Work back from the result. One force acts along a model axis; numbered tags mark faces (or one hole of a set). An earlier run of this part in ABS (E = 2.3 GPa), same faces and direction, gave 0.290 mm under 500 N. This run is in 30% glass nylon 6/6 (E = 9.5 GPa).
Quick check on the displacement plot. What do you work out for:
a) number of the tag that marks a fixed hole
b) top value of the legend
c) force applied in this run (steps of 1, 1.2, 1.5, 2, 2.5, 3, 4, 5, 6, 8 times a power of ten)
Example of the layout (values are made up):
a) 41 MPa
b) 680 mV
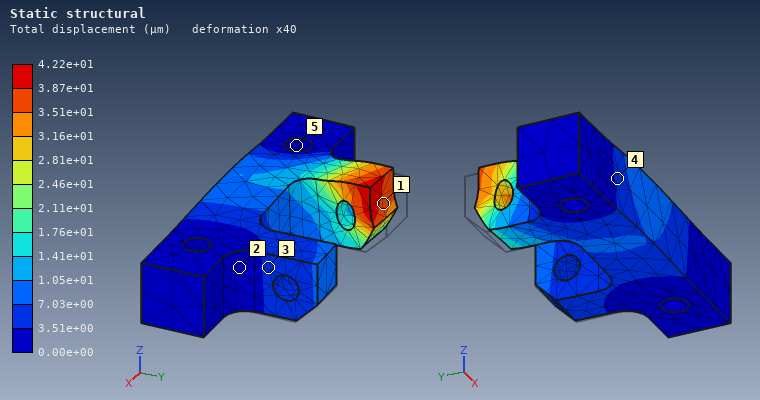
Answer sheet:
a) 5
b) 4.22e+01 µm
c) 300 N
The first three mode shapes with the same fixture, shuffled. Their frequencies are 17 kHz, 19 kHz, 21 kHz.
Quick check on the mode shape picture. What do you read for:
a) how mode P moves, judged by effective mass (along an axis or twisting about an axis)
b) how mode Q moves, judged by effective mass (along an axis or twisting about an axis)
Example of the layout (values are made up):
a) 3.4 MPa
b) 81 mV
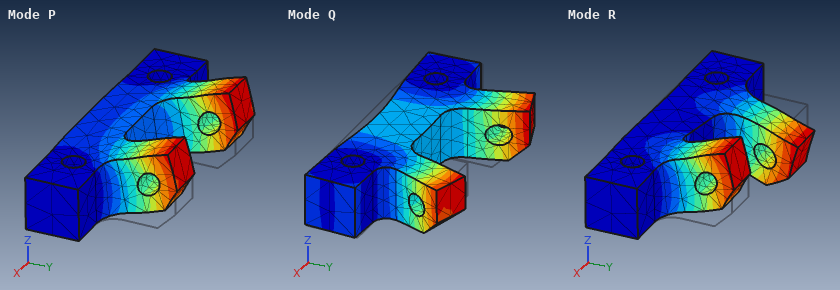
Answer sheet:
a) along Z
b) along Y
